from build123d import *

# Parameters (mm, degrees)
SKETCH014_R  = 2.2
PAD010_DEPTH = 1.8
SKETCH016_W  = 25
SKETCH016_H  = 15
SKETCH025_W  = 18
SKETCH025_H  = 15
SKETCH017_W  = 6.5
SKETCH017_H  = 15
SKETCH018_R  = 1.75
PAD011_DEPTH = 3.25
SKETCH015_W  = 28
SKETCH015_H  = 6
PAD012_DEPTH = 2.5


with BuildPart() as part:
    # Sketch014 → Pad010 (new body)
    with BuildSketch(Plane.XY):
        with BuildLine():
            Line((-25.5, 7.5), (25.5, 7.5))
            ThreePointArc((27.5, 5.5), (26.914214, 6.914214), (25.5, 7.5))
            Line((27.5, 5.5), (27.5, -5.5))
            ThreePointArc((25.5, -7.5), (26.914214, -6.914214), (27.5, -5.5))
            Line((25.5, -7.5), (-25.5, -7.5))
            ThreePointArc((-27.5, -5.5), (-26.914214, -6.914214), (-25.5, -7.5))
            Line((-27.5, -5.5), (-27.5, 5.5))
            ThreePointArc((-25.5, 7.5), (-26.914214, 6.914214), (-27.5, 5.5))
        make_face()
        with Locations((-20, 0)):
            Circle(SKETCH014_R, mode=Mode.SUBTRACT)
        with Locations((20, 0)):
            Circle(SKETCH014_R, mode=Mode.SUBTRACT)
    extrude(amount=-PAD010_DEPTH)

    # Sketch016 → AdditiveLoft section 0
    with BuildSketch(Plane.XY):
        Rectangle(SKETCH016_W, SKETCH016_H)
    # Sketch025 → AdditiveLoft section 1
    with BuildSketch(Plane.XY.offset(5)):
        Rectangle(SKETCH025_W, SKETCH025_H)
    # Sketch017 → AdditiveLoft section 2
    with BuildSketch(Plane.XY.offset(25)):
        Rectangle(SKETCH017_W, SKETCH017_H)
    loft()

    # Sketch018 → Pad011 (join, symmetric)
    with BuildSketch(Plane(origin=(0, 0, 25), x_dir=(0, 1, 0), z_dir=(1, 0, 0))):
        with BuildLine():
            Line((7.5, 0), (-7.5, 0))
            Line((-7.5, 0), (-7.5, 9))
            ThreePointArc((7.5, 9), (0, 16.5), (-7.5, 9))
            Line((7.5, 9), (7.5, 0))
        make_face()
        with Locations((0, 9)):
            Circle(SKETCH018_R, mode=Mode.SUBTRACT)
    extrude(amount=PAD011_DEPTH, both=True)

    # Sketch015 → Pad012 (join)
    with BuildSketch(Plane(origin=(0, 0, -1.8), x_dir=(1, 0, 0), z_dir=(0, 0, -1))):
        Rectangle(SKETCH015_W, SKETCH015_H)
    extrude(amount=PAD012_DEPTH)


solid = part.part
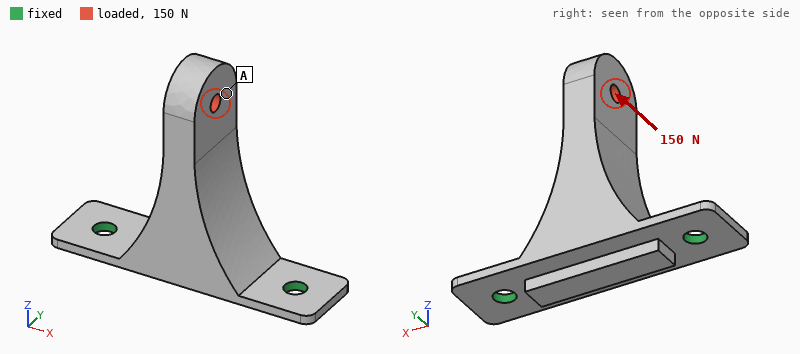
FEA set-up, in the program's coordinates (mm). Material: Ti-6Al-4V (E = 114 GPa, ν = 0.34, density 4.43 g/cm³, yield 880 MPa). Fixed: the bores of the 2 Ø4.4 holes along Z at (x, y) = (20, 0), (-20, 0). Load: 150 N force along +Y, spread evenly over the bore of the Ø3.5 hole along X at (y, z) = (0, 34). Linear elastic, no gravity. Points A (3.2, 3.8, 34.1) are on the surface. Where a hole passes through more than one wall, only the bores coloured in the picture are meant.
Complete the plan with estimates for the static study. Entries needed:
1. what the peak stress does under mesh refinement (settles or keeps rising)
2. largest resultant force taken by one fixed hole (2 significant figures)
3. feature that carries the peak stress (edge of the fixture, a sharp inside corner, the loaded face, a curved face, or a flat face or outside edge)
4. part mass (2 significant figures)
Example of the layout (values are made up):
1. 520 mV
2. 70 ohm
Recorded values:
1. keeps rising
2. 75 N
3. edge of the fixture
4. 35 g
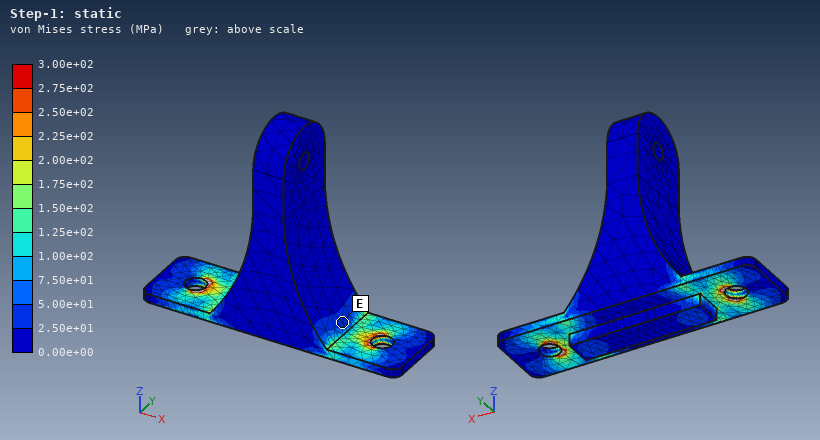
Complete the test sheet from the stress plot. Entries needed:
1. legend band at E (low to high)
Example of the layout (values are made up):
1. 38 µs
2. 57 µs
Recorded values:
1. 2.50e+01 to 5.00e+01 MPa
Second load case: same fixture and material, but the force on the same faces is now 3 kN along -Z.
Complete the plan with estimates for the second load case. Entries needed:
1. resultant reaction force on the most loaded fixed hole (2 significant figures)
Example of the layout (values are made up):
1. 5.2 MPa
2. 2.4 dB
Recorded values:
1. 1.5 kN
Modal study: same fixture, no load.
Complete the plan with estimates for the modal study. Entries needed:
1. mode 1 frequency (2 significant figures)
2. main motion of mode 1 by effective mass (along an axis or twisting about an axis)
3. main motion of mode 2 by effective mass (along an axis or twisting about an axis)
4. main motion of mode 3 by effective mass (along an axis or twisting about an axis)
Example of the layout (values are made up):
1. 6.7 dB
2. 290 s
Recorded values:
1. 1200 Hz
2. along Y
3. along X
4. along Z
